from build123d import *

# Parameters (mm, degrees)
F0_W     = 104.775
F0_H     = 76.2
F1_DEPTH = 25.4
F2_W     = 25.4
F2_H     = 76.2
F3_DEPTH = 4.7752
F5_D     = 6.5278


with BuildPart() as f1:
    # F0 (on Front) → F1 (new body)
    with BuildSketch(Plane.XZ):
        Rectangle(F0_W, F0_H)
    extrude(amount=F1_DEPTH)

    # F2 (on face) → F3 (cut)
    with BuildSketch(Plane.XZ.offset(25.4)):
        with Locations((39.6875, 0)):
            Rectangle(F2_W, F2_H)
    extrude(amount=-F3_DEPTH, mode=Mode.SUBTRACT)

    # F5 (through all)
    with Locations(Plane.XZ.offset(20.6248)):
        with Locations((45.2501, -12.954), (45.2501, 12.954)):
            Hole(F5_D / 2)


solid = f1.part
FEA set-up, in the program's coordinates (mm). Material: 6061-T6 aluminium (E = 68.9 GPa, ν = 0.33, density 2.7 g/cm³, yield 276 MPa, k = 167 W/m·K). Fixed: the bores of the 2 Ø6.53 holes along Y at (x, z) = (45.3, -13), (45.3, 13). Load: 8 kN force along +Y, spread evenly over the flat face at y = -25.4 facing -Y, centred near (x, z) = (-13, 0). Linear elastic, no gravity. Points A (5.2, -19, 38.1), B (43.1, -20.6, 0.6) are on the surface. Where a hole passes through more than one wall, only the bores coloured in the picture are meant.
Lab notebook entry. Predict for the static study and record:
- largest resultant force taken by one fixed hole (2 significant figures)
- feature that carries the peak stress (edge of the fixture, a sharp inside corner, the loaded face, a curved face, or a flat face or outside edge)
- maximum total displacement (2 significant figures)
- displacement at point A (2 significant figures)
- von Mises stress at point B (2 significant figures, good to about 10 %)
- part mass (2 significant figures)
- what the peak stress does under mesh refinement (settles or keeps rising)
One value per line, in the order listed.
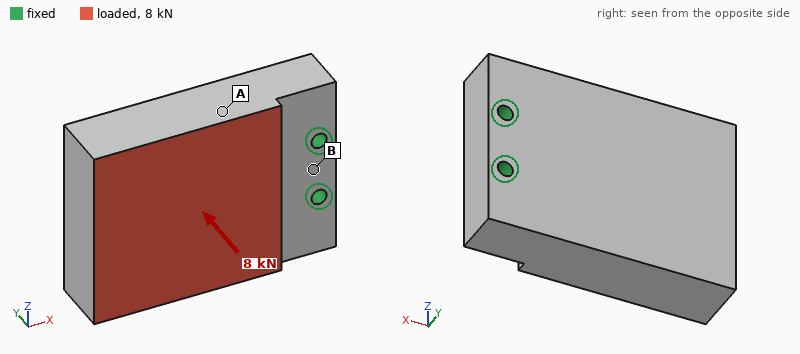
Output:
4.0 kN
edge of the fixture
0.34 mm
0.11 mm
41 MPa
520 g
keeps rising
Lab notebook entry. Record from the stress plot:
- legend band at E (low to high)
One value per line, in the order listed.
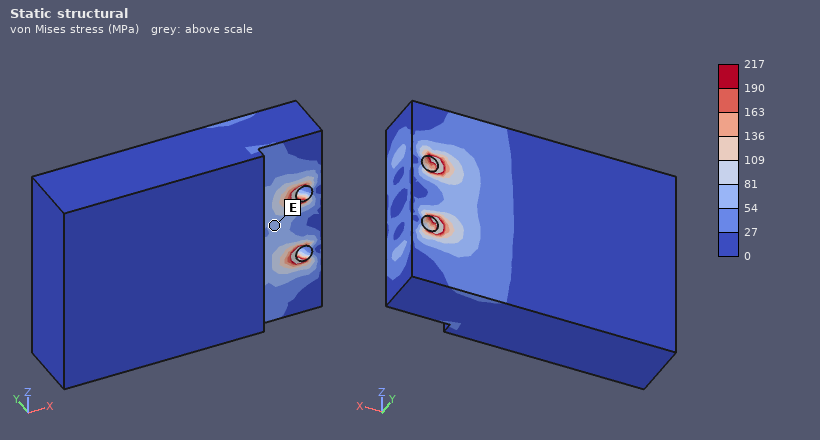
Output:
54 to 81 MPa
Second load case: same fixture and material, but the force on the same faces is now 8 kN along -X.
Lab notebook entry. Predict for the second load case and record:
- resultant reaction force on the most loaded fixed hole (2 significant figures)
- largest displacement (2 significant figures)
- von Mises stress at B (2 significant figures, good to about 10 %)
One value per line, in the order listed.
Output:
4.0 kN
0.11 mm
13 MPa
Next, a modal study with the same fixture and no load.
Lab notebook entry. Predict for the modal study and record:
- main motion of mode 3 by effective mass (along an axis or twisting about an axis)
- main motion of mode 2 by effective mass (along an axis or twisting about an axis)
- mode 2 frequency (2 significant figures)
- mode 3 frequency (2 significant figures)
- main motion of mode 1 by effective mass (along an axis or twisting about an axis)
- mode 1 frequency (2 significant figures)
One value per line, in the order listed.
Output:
twisting about X
along Z
2600 Hz
4000 Hz
along Y
1500 Hz
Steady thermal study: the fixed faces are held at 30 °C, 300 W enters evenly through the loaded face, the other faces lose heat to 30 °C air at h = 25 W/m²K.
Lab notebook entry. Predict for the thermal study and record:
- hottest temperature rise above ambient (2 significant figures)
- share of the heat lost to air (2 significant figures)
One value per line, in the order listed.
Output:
63 K
5.8 %
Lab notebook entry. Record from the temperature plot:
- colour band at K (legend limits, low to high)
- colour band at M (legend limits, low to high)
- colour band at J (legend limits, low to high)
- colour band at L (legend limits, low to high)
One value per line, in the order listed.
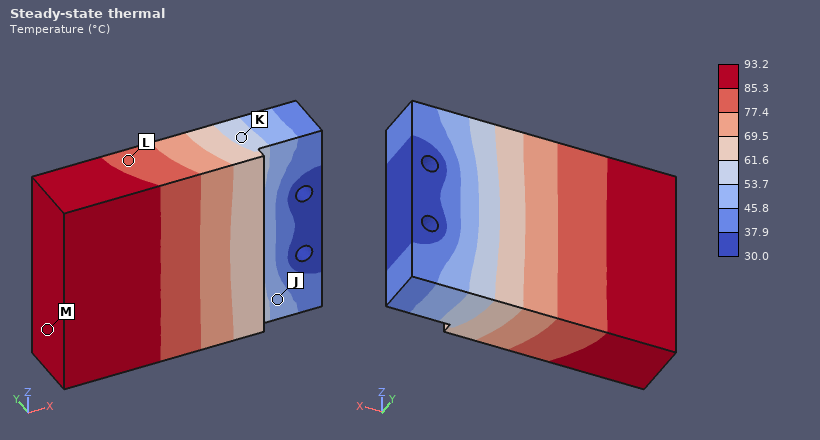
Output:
53.7 to 61.6 °C
85.3 to 93.2 °C
45.8 to 53.7 °C
77.4 to 85.3 °C
